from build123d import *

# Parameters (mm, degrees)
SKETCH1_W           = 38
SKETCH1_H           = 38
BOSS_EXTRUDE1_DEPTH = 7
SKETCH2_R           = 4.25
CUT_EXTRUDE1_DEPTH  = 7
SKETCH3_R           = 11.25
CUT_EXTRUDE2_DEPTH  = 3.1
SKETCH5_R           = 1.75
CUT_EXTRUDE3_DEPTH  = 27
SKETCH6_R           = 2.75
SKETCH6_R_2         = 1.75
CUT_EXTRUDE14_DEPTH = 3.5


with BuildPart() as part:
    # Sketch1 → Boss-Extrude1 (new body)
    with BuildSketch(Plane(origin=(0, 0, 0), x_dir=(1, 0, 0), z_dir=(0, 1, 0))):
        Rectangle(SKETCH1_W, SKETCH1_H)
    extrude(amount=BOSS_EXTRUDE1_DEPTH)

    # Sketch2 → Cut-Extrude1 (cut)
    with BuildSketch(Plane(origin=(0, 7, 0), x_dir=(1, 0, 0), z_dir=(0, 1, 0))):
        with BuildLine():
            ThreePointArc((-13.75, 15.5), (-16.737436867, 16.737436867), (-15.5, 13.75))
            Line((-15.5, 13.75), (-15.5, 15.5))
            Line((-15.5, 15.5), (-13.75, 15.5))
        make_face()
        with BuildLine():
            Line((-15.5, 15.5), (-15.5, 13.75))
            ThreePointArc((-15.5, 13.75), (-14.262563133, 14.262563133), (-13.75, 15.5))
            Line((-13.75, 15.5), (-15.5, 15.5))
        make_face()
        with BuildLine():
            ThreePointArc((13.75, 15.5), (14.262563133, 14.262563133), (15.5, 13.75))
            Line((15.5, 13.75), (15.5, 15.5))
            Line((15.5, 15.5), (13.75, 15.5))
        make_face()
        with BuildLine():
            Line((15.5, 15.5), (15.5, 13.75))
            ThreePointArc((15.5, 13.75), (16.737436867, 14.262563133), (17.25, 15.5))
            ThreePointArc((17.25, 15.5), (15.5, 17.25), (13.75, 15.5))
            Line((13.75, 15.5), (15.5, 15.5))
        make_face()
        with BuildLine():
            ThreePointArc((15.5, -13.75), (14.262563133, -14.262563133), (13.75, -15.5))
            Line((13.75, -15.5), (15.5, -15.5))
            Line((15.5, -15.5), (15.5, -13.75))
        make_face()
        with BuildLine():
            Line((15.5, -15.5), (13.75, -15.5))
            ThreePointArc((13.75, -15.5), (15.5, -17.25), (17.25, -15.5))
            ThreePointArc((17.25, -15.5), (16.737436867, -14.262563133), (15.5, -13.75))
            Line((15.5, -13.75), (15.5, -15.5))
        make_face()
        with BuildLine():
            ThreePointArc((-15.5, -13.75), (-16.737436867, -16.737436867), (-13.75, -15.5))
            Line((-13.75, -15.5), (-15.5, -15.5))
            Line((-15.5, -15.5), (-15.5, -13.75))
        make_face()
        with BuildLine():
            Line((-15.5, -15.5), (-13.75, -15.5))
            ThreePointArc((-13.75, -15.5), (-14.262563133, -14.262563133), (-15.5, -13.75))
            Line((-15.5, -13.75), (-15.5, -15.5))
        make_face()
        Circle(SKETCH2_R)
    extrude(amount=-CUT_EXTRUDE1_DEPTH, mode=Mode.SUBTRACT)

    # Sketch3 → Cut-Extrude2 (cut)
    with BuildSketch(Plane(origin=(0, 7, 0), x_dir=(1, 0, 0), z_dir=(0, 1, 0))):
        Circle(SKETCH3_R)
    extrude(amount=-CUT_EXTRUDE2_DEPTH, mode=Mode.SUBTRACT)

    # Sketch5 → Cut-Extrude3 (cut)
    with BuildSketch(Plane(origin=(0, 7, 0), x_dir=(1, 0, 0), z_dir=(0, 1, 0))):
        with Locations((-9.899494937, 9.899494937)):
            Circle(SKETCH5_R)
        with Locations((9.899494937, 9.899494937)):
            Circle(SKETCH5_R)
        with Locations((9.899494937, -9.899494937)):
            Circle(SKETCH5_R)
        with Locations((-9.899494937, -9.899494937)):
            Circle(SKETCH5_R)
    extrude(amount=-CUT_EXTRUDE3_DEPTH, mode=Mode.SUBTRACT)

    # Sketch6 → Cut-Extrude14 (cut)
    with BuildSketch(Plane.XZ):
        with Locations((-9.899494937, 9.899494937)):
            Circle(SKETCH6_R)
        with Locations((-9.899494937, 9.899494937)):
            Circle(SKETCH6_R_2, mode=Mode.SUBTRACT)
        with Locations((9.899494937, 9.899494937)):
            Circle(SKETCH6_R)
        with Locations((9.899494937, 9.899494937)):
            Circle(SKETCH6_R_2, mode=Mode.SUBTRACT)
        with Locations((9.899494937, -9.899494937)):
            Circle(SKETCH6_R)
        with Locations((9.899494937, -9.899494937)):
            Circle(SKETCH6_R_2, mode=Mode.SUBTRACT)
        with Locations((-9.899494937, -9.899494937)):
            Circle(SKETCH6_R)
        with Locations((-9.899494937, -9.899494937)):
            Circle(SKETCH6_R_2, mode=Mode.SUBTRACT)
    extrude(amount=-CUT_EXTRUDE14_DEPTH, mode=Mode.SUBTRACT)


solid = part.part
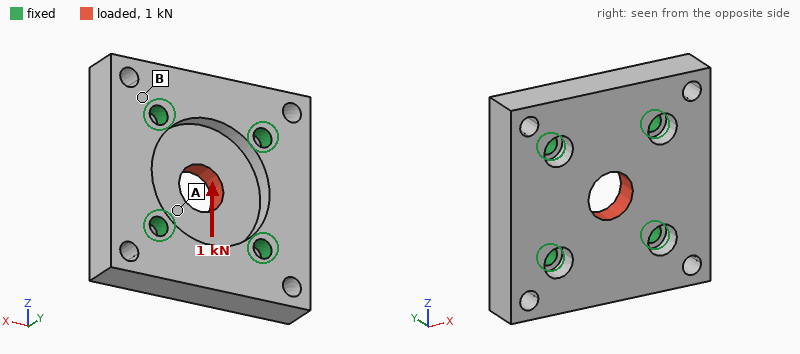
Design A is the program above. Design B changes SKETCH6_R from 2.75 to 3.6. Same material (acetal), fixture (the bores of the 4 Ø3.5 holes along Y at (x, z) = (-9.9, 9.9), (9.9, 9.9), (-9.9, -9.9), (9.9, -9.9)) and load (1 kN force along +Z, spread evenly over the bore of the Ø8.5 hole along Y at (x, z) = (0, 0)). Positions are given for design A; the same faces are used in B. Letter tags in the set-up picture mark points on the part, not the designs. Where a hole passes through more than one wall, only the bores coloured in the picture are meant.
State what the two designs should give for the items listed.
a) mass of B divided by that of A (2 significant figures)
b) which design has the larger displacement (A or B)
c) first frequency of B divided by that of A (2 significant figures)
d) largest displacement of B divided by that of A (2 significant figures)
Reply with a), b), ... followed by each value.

a) 0.97
b) B
c) 0.97
d) 1.1
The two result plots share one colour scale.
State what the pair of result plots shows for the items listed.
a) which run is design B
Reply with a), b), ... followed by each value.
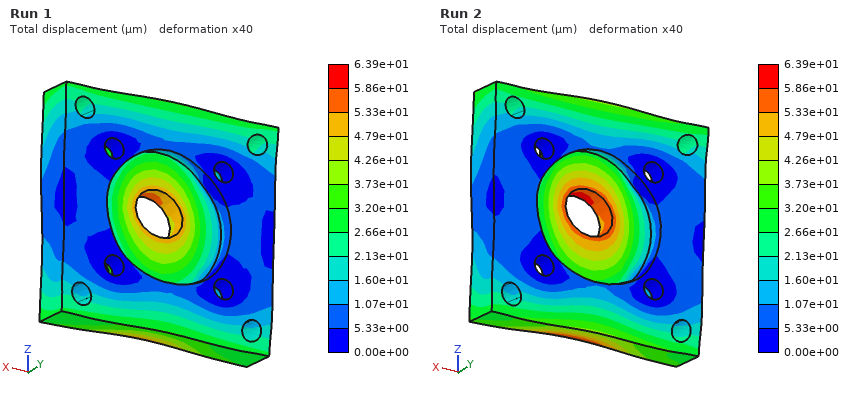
a) Run 2
